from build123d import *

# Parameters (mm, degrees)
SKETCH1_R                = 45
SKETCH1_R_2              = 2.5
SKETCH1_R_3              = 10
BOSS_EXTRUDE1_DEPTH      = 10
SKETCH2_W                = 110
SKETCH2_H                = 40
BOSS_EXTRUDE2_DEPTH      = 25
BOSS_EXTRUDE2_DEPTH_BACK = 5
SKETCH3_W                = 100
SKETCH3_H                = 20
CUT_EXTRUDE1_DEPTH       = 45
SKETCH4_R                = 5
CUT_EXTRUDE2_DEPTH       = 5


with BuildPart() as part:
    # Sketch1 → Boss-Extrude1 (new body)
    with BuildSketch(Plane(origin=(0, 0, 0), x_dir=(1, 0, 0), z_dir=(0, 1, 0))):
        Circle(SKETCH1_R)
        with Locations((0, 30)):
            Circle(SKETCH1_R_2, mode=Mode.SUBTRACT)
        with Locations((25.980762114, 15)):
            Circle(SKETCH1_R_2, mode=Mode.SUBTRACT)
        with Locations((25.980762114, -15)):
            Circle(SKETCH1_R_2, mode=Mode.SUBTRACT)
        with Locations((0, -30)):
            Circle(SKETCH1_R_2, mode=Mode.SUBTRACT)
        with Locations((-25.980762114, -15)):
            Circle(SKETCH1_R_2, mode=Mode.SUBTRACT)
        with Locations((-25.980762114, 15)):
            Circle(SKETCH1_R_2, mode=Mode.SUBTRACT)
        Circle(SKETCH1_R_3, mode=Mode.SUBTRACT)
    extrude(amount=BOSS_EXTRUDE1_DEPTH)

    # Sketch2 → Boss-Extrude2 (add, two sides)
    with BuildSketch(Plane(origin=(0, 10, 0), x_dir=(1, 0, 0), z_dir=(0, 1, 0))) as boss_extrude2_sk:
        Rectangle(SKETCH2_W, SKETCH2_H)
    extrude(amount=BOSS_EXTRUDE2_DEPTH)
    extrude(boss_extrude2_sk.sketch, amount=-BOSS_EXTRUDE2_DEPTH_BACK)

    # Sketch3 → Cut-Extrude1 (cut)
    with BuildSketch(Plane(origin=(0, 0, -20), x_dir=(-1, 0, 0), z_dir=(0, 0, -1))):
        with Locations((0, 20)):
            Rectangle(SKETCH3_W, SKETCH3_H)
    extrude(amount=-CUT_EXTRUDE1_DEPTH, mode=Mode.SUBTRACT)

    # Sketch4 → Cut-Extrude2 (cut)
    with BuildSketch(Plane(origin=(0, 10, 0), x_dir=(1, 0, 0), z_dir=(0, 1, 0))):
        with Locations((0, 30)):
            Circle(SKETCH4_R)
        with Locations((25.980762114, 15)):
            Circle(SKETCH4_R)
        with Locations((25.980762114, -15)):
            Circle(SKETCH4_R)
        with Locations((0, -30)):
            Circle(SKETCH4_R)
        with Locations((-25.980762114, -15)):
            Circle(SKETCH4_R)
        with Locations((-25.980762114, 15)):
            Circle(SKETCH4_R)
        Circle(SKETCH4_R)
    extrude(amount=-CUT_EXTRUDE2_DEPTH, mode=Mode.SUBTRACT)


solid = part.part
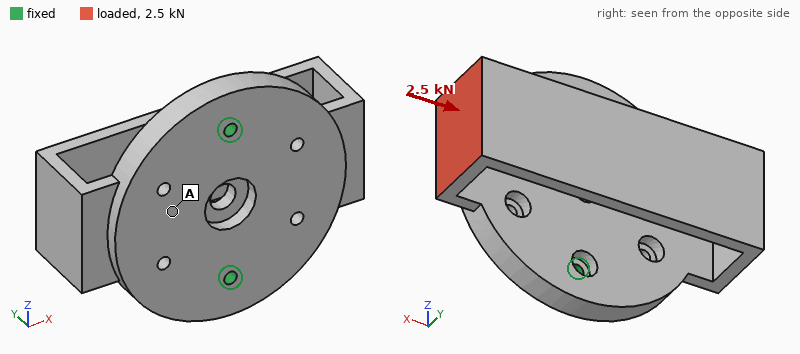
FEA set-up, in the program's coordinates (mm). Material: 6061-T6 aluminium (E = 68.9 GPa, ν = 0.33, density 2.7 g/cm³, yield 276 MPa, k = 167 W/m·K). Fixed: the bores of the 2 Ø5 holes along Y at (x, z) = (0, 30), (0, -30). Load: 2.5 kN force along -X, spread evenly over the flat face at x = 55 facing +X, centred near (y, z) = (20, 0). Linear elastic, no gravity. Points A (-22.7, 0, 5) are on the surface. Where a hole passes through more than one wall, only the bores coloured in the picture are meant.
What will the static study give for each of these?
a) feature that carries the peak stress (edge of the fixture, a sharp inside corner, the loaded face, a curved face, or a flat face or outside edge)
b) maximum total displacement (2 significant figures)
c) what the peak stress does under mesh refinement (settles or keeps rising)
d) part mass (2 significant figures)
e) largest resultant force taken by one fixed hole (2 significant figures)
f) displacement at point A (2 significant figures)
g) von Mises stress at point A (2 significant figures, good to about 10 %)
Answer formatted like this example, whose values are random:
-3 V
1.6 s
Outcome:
edge of the fixture
0.38 mm
keeps rising
250 g
1.3 kN
0.078 mm
14 MPa
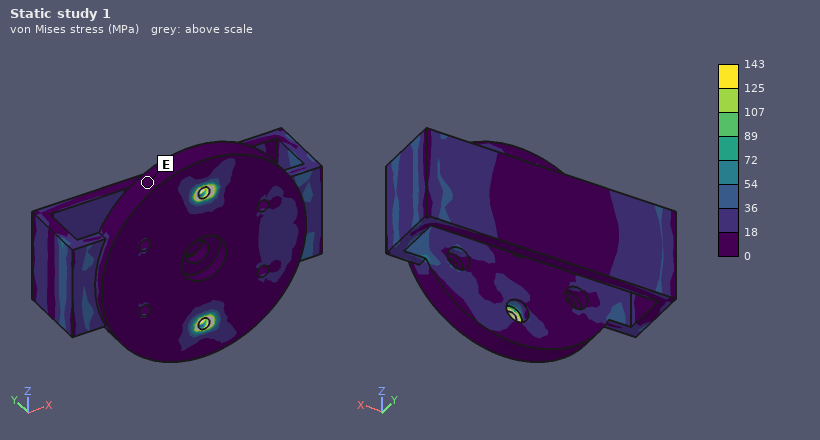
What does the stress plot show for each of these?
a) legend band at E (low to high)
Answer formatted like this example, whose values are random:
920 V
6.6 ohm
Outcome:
0 to 18 MPa
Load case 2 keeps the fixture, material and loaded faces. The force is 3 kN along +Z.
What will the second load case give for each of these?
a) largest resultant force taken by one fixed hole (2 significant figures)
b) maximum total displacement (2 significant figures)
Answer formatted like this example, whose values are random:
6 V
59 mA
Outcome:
3.2 kN
0.20 mm
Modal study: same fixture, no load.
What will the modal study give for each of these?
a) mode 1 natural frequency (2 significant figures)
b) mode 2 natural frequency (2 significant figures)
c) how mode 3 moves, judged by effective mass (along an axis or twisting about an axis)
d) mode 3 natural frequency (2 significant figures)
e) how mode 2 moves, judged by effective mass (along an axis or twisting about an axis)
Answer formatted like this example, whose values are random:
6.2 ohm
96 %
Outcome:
960 Hz
1500 Hz
along Z
2200 Hz
along Y
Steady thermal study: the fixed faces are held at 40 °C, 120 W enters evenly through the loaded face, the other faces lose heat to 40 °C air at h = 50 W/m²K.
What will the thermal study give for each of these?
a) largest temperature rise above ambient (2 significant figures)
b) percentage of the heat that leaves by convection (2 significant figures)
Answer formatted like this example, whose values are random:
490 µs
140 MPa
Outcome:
86 K
37 %
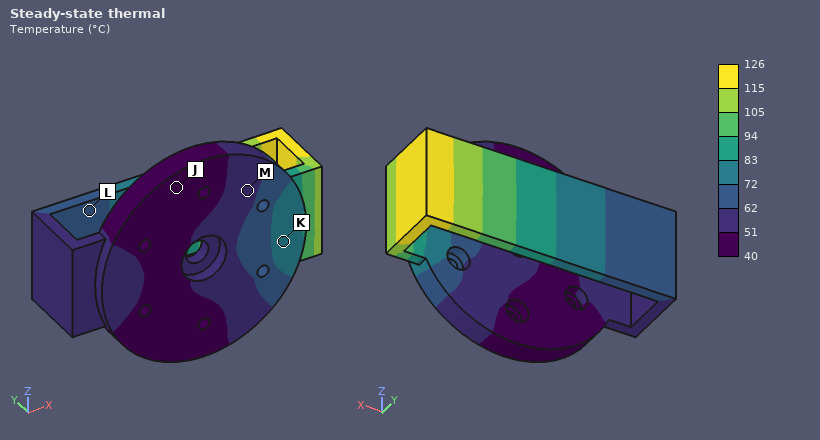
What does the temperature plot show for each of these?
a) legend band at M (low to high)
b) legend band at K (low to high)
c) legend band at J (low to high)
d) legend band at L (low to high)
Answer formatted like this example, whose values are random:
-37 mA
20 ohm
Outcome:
51 to 62 °C
72 to 83 °C
40 to 51 °C
62 to 72 °C
